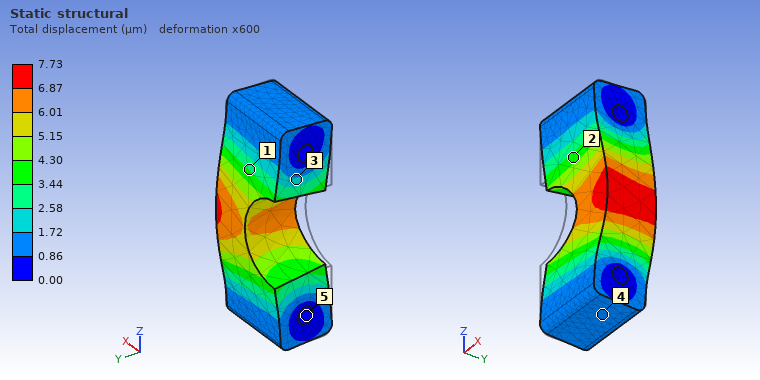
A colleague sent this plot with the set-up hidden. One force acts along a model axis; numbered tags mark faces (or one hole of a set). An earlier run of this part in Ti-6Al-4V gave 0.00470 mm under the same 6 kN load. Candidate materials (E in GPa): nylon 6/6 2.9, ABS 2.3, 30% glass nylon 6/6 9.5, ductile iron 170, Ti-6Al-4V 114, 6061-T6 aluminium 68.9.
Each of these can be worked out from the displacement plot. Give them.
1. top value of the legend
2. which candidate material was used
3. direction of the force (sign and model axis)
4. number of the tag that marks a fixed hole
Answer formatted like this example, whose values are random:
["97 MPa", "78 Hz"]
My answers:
["7.73 µm", "6061-T6 aluminium", "+Y", "5"]
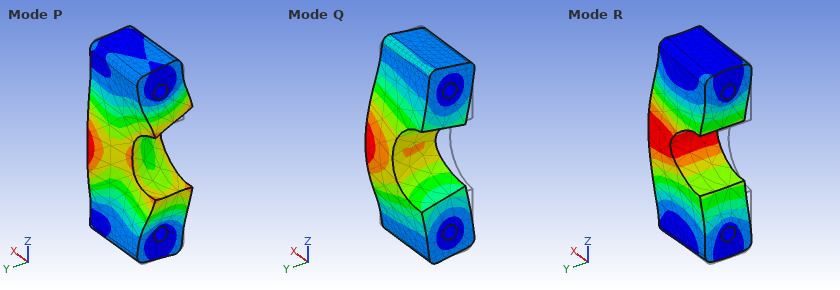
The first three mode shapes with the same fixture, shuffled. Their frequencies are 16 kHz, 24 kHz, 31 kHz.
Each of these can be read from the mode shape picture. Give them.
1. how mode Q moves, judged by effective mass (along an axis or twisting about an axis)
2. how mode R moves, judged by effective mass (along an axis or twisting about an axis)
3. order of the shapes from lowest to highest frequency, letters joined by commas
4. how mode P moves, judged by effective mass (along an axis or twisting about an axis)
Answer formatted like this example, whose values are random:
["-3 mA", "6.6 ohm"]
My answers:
["along Y", "along X", "Q, R, P", "twisting about Z"]
